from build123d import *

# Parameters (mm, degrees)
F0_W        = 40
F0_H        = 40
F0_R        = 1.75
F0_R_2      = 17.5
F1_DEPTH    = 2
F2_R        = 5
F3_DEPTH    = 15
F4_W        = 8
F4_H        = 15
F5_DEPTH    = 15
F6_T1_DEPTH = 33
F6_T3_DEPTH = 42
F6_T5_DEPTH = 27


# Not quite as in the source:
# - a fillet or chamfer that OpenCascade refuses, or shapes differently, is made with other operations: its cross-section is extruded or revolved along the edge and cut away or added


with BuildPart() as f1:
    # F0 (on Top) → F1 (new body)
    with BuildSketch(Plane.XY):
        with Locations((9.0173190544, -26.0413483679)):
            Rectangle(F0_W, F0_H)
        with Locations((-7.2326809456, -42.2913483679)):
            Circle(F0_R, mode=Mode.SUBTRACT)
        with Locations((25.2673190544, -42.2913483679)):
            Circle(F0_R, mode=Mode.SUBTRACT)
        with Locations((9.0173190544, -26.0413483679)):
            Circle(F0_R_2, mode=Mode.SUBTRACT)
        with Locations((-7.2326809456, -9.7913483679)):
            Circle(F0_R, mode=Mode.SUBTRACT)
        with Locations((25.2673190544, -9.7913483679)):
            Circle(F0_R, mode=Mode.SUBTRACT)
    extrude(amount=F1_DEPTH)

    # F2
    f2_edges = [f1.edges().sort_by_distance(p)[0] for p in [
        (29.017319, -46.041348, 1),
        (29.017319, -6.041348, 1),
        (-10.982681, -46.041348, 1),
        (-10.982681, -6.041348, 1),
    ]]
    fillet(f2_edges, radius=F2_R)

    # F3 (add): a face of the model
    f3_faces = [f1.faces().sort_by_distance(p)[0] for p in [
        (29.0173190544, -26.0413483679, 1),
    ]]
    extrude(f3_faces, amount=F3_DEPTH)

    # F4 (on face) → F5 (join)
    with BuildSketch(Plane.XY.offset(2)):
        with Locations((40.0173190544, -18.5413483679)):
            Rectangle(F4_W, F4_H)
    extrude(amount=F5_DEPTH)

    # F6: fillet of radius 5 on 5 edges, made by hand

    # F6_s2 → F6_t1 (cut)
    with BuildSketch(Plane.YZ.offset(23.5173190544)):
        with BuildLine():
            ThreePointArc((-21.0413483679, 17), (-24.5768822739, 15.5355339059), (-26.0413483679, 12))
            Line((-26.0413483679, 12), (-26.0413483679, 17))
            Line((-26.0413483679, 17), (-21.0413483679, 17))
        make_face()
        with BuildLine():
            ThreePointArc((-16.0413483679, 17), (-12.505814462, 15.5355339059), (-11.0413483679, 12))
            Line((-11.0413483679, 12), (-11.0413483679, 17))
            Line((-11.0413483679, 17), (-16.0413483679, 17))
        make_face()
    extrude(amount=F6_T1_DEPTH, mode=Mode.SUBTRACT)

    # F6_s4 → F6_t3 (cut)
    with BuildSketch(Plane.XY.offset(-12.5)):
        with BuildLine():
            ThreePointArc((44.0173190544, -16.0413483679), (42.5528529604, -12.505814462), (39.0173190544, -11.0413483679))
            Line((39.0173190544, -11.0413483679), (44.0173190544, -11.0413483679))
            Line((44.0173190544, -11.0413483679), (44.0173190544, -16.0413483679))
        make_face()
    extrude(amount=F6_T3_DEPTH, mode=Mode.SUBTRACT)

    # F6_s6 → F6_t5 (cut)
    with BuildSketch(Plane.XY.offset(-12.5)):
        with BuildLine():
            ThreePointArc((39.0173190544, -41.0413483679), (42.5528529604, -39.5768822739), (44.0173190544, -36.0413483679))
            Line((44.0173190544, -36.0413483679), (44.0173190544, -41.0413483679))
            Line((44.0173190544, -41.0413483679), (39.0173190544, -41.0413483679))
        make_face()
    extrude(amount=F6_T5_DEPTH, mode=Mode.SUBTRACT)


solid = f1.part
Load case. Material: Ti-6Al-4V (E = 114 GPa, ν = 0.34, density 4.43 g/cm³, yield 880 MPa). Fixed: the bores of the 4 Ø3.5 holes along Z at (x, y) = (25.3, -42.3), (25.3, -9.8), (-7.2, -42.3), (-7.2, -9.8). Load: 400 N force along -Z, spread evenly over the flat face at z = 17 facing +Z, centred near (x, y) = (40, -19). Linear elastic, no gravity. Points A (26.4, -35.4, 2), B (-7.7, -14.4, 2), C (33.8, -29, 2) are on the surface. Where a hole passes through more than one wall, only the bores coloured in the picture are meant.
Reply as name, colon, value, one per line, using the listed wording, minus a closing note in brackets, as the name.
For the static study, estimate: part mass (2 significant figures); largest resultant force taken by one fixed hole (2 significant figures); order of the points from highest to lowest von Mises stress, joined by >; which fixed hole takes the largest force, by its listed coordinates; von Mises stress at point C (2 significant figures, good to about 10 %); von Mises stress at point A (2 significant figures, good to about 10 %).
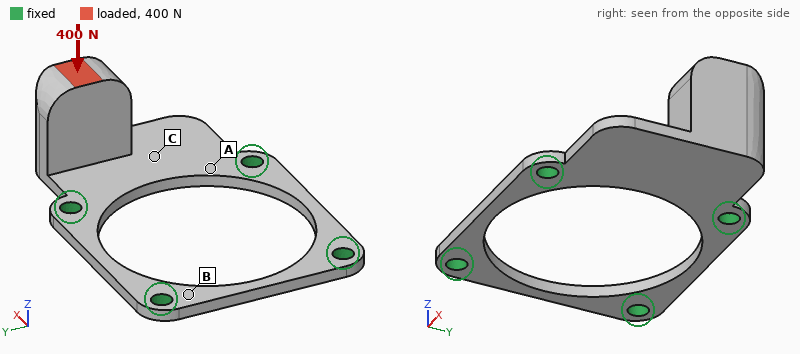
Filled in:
part mass: 16 g
largest resultant force taken by one fixed hole: 310 N
order of the points from highest to lowest von Mises stress, joined by >: A > C > B
which fixed hole takes the largest force, by its listed coordinates: (25.3, -9.8)
von Mises stress at point C: 130 MPa
von Mises stress at point A: 280 MPa
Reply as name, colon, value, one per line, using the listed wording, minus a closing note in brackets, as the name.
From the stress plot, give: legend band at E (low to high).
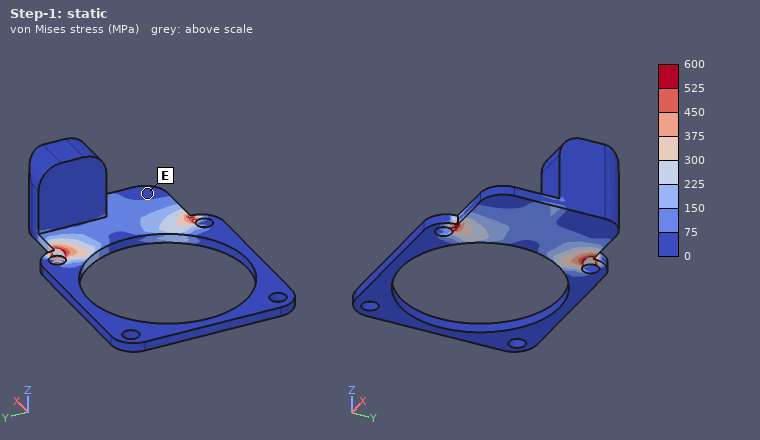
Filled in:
legend band at E: 0 to 75 MPa
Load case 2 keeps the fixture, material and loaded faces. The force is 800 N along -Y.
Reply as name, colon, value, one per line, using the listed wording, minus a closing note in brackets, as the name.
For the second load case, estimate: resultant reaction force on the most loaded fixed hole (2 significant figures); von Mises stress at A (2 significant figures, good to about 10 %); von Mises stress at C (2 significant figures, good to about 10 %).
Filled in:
resultant reaction force on the most loaded fixed hole: 760 N
von Mises stress at A: 140 MPa
von Mises stress at C: 330 MPa
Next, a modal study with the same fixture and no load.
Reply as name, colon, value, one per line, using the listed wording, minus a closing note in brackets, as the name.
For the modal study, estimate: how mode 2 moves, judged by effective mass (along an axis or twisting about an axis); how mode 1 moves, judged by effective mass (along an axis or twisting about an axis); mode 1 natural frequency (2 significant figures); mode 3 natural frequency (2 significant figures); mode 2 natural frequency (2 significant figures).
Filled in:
how mode 2 moves, judged by effective mass: along Y
how mode 1 moves, judged by effective mass: along Z
mode 1 natural frequency: 1400 Hz
mode 3 natural frequency: 5900 Hz
mode 2 natural frequency: 3800 Hz
